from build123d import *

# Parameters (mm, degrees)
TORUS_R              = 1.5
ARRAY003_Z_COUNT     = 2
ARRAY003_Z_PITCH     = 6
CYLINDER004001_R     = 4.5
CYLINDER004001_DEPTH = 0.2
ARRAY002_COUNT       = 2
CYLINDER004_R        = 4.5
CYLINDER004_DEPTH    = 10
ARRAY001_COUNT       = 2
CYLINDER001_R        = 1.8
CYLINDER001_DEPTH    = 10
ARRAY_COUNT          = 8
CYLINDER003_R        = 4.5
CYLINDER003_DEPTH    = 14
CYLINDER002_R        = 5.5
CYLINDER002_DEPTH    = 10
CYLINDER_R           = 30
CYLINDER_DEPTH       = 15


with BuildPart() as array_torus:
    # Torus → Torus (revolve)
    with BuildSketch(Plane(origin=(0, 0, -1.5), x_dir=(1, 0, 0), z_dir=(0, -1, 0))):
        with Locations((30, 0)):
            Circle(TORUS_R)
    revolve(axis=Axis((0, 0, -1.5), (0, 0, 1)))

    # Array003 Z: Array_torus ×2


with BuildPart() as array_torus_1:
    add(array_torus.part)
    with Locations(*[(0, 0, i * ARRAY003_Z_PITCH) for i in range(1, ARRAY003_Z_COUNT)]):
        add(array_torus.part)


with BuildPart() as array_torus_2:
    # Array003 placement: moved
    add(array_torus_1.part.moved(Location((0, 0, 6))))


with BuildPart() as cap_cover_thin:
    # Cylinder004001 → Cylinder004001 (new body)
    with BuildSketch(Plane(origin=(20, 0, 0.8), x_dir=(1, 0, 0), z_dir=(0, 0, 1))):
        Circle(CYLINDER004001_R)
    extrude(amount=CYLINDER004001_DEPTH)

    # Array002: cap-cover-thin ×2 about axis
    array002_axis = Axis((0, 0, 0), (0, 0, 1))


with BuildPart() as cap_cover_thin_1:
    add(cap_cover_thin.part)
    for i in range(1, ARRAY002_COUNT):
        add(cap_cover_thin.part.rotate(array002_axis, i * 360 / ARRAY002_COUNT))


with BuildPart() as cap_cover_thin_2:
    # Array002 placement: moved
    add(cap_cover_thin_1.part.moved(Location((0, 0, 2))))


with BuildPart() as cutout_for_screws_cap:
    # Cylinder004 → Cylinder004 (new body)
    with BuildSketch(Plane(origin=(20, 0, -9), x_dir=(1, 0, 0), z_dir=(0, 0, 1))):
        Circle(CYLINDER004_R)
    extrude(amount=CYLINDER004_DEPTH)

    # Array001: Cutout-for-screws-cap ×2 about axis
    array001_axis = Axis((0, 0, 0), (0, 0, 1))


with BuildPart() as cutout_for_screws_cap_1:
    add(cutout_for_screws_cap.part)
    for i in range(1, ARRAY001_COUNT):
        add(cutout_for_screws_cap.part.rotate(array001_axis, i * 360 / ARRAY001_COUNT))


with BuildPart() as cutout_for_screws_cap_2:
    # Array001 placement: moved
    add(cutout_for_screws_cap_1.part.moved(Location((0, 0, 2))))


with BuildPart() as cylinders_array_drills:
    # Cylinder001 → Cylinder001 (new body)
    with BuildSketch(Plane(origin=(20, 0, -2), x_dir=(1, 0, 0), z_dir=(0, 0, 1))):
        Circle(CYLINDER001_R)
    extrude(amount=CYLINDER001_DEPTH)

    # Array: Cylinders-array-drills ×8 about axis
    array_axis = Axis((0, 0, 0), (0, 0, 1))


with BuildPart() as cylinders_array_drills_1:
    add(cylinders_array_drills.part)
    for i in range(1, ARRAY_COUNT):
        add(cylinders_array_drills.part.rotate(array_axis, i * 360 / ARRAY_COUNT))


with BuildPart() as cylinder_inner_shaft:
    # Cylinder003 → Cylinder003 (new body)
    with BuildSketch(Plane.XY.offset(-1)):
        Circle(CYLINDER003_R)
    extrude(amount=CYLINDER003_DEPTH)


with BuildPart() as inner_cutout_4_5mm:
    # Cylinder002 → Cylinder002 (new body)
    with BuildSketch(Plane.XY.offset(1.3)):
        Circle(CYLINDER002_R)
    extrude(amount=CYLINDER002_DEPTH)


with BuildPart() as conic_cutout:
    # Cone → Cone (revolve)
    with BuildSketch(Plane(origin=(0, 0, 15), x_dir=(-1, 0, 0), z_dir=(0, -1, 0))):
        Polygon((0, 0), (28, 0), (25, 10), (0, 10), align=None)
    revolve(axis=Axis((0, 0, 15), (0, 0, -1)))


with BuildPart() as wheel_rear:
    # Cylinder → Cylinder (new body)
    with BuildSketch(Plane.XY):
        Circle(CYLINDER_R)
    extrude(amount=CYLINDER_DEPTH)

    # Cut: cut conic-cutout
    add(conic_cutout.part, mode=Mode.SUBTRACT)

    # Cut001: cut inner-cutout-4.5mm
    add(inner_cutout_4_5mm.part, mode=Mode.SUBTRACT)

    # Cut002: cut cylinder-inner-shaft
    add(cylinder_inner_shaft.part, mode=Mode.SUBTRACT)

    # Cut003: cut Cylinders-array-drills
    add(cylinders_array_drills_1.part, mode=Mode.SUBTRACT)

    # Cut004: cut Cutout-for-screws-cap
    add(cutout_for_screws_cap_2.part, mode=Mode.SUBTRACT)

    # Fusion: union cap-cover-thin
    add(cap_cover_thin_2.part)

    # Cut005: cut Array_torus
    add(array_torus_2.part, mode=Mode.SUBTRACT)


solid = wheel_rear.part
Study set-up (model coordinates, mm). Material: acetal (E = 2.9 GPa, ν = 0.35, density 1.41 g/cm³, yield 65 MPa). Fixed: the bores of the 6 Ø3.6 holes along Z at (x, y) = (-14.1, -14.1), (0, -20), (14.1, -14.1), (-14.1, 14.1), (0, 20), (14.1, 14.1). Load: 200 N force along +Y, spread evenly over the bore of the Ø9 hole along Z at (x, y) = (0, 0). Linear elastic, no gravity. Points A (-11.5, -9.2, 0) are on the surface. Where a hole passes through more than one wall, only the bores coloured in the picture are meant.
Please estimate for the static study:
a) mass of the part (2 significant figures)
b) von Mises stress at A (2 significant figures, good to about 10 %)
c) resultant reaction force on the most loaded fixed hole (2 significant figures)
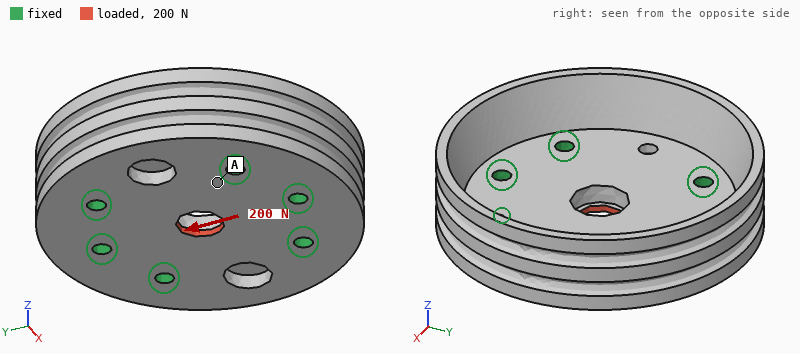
25 g
0.76 MPa
44 N
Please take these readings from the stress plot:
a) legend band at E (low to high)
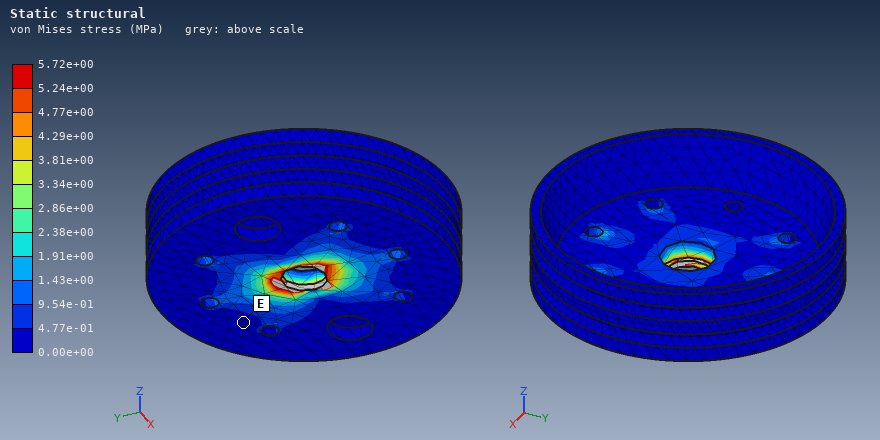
0.00e+00 to 4.77e-01 MPa
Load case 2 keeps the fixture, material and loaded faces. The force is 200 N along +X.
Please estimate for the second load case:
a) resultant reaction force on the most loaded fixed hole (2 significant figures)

47 N
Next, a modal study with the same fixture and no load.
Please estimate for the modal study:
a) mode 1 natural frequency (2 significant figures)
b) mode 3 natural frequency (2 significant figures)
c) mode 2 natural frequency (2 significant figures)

3500 Hz
4900 Hz
3800 Hz
